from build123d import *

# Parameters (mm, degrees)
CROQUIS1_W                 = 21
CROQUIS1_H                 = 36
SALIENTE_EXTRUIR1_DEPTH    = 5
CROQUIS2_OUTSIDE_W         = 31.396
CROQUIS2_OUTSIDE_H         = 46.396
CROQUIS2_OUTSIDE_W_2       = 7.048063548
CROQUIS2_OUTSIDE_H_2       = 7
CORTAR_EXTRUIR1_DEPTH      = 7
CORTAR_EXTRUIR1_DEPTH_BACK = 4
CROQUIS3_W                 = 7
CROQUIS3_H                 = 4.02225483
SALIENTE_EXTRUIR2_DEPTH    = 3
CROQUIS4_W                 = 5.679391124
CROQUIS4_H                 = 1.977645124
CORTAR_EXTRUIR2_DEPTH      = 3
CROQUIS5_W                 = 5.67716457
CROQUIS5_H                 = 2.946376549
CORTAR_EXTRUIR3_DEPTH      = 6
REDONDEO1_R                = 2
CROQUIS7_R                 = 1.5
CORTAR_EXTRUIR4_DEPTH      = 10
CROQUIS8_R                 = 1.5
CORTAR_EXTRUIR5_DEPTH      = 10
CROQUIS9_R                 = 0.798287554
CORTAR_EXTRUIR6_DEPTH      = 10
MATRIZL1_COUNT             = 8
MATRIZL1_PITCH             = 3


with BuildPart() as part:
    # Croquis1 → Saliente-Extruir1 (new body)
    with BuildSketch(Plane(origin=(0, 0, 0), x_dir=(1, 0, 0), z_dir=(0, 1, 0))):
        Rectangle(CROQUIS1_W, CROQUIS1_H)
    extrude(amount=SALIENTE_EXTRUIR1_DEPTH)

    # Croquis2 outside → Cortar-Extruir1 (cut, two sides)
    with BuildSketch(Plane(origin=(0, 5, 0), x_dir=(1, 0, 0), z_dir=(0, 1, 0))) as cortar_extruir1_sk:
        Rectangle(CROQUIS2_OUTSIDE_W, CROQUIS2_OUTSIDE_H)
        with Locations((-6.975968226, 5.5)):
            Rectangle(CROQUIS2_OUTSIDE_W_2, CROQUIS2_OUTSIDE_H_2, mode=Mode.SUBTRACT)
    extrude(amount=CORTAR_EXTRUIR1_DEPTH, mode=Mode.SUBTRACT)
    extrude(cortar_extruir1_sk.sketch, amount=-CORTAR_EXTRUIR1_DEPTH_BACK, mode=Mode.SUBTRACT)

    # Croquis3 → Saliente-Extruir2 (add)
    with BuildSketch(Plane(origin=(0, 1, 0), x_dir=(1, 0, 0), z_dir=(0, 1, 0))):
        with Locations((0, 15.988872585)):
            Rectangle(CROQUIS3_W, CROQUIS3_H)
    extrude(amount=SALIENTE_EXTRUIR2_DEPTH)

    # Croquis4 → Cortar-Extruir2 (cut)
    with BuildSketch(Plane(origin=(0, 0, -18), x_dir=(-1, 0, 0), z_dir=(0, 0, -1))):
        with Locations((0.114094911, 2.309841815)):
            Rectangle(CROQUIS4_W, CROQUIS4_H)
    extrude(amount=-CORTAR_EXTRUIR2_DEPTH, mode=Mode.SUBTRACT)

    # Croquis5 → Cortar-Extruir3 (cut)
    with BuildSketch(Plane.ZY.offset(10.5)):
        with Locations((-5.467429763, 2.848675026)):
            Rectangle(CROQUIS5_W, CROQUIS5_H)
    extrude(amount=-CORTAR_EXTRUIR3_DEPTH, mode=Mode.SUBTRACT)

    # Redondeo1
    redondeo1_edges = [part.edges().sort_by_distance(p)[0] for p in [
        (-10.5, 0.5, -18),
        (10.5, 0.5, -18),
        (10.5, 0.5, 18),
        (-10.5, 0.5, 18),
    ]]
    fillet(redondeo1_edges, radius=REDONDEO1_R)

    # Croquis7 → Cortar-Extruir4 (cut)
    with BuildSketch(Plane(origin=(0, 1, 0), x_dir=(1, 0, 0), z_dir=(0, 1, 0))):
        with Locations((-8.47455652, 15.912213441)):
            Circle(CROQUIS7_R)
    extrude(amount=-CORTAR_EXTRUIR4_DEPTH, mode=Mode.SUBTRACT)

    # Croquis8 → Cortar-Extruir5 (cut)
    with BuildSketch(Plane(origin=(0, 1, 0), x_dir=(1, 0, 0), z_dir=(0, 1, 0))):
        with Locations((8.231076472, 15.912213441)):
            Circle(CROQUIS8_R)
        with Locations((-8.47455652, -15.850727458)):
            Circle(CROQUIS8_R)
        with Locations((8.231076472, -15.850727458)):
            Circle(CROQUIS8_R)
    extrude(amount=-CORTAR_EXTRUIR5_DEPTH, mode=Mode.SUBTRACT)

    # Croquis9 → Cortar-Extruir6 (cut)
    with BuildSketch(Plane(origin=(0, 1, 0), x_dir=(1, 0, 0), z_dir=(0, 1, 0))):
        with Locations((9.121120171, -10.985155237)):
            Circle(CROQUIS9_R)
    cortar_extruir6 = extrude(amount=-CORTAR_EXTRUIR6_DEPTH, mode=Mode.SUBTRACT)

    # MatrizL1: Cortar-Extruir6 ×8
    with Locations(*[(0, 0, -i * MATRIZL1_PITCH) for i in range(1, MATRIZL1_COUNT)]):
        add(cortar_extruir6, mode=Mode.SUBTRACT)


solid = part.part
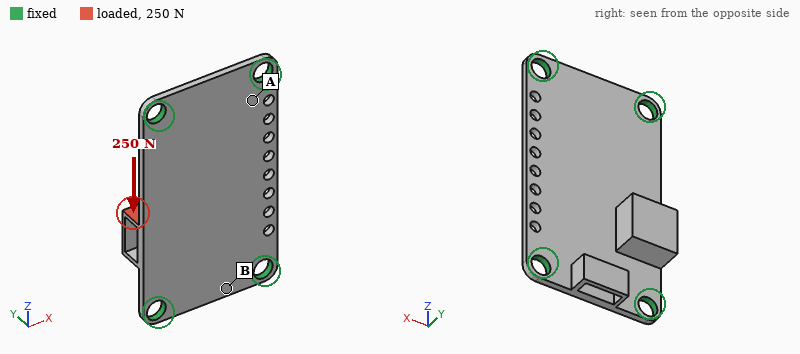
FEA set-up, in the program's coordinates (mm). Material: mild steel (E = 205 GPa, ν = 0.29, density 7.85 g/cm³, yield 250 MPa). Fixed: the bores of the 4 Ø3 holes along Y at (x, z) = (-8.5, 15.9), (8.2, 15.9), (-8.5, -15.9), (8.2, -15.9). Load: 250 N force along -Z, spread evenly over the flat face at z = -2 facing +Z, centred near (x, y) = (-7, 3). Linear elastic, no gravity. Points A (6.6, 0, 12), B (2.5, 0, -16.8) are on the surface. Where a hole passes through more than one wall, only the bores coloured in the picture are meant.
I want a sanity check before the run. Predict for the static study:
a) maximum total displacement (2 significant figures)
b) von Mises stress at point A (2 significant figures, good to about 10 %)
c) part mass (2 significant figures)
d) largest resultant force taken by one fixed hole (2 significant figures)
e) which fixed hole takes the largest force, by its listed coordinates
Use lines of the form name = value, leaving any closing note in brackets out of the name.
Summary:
maximum total displacement = 31 µm
von Mises stress at point A = 29 MPa
part mass = 6.7 g
largest resultant force taken by one fixed hole = 120 N
which fixed hole takes the largest force, by its listed coordinates = (-8.5, -15.9)
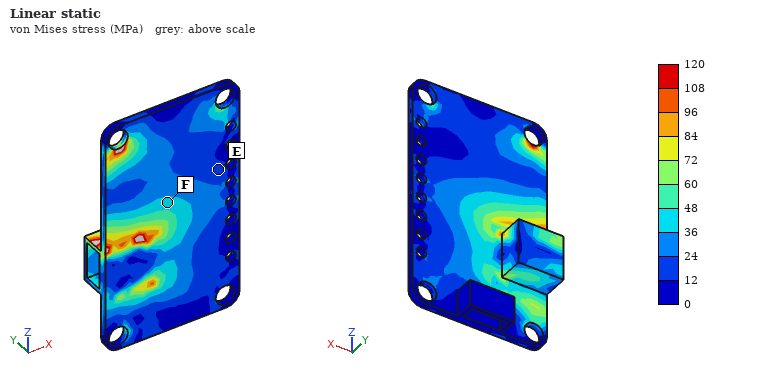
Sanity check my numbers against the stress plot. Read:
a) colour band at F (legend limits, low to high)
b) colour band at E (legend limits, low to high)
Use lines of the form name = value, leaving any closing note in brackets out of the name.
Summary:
colour band at F = 36 to 48 MPa
colour band at E = 12 to 24 MPa
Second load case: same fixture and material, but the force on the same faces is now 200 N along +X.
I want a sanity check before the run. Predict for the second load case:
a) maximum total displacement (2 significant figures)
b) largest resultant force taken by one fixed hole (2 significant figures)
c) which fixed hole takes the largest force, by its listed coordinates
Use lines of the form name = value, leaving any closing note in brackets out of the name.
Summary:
maximum total displacement = 31 µm
largest resultant force taken by one fixed hole = 98 N
which fixed hole takes the largest force, by its listed coordinates = (8.2, -15.9)
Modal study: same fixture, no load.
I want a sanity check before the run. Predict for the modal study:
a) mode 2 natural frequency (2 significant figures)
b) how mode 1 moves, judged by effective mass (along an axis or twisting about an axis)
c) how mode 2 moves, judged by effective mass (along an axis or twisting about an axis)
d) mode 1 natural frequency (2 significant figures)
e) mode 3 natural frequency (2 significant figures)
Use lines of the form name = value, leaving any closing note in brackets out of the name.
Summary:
mode 2 natural frequency = 8000 Hz
how mode 1 moves, judged by effective mass = along Y
how mode 2 moves, judged by effective mass = twisting about Z
mode 1 natural frequency = 5100 Hz
mode 3 natural frequency = 14 kHz
